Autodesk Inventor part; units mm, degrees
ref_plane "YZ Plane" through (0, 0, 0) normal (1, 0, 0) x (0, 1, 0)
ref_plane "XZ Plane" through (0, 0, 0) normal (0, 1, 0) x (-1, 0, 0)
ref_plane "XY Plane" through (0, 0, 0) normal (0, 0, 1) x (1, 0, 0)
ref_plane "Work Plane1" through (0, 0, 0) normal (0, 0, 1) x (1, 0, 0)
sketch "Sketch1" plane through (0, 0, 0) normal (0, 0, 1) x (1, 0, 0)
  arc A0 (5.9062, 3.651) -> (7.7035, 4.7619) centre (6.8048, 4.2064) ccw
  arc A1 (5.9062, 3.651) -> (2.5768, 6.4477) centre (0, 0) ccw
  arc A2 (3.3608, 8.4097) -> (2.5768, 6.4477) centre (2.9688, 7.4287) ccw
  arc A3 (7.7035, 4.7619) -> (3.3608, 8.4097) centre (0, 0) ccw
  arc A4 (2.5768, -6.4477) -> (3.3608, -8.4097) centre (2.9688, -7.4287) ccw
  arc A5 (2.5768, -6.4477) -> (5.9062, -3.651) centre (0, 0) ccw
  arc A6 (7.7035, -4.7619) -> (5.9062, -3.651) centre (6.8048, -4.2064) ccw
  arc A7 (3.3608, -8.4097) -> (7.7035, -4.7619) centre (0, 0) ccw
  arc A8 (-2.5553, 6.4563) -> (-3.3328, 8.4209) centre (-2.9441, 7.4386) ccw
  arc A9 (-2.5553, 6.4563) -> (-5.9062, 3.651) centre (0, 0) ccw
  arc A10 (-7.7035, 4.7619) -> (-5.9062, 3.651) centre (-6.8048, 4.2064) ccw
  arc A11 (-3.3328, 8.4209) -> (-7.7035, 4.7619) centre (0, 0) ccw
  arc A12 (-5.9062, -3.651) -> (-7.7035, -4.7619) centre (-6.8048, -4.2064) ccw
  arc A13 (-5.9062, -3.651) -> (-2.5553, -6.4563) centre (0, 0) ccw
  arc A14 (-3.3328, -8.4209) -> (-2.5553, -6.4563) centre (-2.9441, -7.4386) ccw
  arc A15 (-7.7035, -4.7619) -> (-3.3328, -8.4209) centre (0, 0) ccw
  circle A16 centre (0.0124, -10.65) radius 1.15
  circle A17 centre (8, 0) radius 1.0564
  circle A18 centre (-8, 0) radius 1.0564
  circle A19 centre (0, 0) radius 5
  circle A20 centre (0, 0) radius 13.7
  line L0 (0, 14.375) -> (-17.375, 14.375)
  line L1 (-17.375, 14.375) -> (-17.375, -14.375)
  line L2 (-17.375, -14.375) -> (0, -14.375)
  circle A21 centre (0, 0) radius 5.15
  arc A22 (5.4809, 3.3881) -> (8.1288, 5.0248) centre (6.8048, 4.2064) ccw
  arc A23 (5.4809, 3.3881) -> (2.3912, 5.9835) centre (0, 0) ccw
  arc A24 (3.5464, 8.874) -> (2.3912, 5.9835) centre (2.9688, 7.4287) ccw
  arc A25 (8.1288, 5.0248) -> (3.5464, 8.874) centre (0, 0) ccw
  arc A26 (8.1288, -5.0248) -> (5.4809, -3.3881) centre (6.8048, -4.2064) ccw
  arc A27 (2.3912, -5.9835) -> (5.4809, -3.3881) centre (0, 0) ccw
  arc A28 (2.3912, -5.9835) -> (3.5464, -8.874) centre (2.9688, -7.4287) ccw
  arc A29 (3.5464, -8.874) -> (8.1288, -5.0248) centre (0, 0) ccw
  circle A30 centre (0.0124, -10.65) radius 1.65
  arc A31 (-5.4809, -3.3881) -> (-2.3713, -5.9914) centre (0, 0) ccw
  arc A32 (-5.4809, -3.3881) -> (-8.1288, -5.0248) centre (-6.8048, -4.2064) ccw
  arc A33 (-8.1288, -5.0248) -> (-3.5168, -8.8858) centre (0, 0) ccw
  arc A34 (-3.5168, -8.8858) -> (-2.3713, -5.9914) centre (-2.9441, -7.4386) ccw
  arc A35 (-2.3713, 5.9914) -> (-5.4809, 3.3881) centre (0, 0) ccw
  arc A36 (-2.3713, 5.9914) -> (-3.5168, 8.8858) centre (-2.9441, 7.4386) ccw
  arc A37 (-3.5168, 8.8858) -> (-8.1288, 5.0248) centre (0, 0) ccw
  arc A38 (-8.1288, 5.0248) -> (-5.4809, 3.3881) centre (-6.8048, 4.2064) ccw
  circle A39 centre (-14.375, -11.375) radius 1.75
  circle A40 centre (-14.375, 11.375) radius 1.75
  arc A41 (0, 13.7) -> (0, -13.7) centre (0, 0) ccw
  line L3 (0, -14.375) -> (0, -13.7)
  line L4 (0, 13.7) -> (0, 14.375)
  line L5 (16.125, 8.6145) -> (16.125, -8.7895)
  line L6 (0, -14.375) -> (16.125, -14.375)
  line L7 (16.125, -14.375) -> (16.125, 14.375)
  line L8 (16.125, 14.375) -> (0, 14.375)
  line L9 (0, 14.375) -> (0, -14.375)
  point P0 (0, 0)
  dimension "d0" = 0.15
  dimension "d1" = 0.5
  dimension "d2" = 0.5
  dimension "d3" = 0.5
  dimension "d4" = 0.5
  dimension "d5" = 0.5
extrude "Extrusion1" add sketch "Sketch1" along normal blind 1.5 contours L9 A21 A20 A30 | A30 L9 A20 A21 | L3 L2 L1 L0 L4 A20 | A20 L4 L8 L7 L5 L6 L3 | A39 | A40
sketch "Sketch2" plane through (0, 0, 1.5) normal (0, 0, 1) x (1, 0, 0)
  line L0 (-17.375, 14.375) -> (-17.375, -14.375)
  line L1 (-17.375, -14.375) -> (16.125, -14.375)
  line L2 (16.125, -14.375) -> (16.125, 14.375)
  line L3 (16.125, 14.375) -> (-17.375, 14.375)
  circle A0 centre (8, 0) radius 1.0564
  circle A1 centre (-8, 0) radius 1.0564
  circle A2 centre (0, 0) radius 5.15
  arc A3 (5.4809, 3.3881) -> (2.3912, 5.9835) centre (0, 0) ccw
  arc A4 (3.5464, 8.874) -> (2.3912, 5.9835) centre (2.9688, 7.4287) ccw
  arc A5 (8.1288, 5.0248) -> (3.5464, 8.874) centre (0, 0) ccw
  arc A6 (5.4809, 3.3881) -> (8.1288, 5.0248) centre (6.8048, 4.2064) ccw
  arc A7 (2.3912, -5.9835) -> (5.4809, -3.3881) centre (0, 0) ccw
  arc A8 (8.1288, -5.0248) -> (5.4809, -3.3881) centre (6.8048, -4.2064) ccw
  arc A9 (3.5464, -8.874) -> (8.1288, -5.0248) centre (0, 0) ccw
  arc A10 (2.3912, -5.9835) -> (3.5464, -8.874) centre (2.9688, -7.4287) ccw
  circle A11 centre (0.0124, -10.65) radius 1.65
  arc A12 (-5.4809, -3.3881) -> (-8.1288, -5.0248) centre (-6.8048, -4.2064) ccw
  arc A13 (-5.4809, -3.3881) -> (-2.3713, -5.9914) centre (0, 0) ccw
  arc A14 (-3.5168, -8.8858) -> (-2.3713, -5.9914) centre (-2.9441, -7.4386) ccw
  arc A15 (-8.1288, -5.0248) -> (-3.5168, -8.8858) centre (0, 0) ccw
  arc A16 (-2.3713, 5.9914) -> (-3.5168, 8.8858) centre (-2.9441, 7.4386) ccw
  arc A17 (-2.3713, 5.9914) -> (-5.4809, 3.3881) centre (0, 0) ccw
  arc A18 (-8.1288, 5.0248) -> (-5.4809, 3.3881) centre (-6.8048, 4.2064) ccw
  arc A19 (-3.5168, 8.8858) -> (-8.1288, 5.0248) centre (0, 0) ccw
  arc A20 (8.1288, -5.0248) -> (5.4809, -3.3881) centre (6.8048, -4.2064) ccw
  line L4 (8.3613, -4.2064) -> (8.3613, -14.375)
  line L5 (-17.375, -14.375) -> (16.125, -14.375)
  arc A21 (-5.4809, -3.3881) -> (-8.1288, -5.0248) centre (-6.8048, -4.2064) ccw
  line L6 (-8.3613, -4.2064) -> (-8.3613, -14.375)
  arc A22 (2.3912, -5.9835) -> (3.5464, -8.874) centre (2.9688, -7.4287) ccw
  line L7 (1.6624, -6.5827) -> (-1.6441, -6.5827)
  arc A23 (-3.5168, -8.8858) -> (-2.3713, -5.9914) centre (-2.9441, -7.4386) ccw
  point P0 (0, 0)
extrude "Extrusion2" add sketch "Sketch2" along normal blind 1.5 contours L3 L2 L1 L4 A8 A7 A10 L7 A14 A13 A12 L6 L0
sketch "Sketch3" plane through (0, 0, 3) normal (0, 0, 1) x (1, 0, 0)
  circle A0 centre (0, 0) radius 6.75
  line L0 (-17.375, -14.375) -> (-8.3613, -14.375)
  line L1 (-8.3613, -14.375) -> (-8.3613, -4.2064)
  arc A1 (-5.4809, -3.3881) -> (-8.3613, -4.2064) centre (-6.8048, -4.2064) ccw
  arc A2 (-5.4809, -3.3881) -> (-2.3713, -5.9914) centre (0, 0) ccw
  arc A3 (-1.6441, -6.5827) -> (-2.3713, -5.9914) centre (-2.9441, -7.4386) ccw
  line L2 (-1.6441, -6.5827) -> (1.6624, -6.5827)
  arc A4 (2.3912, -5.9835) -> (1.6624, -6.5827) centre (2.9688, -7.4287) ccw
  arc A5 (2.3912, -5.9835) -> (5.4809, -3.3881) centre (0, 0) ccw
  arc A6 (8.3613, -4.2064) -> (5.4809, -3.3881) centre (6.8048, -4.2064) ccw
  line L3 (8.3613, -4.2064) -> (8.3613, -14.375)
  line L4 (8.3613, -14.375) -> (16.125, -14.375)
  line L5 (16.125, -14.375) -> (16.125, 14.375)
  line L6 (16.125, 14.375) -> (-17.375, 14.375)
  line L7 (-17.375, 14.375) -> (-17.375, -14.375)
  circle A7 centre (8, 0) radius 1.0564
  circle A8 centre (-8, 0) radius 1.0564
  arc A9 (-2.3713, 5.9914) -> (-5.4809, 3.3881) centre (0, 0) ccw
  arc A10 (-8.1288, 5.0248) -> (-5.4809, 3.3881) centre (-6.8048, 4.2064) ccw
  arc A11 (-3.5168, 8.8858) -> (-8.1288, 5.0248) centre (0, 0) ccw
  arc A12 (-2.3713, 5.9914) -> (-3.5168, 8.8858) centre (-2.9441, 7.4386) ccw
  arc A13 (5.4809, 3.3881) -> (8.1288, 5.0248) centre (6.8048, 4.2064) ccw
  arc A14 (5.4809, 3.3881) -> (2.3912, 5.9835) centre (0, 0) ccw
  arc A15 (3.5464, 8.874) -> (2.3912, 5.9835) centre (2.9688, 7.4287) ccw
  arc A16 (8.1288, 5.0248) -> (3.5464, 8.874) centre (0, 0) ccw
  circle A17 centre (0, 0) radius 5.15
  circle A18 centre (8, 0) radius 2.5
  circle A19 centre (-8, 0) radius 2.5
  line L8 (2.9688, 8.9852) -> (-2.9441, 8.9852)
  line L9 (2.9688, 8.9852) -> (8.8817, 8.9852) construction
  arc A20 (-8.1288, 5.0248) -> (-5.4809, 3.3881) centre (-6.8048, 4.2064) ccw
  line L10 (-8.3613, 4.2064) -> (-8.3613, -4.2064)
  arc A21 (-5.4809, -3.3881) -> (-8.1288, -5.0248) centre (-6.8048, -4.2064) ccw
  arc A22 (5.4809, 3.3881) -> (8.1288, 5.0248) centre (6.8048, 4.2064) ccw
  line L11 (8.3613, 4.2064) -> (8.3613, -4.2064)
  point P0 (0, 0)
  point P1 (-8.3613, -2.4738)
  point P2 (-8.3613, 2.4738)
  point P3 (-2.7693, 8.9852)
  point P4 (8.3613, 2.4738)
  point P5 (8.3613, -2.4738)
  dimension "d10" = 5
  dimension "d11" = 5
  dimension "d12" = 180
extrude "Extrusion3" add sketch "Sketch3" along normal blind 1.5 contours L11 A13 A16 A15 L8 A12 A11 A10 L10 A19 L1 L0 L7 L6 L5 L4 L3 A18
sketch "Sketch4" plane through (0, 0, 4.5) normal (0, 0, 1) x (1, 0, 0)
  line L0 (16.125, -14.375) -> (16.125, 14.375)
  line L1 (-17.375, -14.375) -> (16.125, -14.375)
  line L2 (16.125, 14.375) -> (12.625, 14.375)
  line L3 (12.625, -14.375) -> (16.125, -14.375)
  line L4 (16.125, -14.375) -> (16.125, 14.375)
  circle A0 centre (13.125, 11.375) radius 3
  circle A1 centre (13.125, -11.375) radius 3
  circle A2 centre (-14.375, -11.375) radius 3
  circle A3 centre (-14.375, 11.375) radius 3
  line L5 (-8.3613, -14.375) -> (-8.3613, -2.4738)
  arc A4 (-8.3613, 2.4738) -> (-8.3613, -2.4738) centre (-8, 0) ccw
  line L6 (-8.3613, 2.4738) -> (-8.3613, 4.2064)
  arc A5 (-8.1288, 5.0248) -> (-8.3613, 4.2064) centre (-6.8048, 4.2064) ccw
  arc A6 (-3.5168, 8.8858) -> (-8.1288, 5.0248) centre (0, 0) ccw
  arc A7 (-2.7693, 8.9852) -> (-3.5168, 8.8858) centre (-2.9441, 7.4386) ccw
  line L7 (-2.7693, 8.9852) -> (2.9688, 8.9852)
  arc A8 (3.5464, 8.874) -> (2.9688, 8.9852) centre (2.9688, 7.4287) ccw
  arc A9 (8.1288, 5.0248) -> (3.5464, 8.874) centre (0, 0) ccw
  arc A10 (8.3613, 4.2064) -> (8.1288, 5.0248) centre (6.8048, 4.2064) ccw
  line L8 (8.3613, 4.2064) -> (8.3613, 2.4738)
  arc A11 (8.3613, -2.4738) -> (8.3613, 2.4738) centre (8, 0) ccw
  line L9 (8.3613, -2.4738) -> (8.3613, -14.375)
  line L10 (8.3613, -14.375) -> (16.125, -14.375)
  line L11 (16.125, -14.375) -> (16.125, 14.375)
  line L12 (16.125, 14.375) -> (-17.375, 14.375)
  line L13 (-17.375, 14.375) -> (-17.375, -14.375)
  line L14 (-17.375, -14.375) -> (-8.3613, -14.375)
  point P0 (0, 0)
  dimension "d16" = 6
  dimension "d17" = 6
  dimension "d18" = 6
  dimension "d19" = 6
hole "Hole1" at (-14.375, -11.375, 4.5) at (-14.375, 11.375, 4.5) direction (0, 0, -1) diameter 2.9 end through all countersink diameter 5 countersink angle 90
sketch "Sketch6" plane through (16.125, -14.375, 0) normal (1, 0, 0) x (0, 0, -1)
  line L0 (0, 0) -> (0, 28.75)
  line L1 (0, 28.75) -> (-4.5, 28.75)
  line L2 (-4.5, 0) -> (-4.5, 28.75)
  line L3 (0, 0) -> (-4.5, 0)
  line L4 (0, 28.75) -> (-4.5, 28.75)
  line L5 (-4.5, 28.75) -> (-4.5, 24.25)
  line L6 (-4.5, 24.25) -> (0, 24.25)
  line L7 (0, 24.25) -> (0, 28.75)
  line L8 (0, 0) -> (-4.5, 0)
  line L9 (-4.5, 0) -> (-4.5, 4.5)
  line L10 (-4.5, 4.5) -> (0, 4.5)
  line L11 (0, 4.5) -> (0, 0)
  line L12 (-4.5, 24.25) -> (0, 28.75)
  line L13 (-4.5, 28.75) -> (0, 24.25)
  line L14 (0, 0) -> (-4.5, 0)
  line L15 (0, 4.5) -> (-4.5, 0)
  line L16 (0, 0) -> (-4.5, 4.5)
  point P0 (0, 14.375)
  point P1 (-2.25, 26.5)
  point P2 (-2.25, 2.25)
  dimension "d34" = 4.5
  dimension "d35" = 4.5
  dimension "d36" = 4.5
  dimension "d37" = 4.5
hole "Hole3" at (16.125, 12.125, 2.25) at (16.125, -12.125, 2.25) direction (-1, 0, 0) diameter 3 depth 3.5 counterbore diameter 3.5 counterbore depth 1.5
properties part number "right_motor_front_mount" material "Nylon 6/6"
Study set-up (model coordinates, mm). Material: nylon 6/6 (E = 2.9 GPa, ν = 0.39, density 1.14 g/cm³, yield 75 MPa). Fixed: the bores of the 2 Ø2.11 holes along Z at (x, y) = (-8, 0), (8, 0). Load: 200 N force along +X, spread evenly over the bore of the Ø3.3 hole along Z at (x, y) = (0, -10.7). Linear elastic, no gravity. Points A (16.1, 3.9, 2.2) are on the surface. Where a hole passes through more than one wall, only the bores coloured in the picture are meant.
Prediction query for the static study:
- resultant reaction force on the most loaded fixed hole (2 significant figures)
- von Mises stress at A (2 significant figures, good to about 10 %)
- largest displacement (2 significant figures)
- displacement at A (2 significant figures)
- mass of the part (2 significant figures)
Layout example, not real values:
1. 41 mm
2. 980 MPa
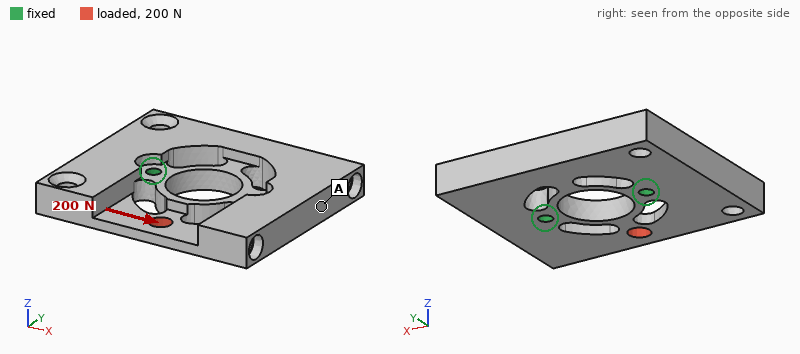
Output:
1. 150 N
2. 4.8 MPa
3. 0.15 mm
4. 0.054 mm
5. 3.3 g
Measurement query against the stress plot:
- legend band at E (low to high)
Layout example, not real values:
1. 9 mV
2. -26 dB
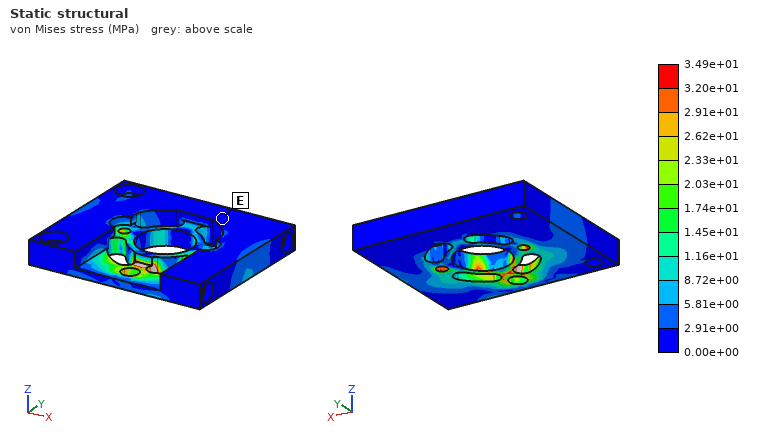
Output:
1. 0.00e+00 to 2.91e+00 MPa
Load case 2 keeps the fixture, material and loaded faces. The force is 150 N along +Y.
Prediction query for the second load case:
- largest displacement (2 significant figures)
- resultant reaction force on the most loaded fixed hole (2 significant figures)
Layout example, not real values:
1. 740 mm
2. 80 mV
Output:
1. 0.13 mm
2. 98 N
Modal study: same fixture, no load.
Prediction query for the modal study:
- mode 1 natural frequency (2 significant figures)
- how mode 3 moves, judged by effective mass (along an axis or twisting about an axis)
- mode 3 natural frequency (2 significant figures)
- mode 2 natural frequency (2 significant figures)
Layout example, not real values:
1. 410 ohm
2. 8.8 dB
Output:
1. 2300 Hz
2. along Z
3. 4100 Hz
4. 3400 Hz
